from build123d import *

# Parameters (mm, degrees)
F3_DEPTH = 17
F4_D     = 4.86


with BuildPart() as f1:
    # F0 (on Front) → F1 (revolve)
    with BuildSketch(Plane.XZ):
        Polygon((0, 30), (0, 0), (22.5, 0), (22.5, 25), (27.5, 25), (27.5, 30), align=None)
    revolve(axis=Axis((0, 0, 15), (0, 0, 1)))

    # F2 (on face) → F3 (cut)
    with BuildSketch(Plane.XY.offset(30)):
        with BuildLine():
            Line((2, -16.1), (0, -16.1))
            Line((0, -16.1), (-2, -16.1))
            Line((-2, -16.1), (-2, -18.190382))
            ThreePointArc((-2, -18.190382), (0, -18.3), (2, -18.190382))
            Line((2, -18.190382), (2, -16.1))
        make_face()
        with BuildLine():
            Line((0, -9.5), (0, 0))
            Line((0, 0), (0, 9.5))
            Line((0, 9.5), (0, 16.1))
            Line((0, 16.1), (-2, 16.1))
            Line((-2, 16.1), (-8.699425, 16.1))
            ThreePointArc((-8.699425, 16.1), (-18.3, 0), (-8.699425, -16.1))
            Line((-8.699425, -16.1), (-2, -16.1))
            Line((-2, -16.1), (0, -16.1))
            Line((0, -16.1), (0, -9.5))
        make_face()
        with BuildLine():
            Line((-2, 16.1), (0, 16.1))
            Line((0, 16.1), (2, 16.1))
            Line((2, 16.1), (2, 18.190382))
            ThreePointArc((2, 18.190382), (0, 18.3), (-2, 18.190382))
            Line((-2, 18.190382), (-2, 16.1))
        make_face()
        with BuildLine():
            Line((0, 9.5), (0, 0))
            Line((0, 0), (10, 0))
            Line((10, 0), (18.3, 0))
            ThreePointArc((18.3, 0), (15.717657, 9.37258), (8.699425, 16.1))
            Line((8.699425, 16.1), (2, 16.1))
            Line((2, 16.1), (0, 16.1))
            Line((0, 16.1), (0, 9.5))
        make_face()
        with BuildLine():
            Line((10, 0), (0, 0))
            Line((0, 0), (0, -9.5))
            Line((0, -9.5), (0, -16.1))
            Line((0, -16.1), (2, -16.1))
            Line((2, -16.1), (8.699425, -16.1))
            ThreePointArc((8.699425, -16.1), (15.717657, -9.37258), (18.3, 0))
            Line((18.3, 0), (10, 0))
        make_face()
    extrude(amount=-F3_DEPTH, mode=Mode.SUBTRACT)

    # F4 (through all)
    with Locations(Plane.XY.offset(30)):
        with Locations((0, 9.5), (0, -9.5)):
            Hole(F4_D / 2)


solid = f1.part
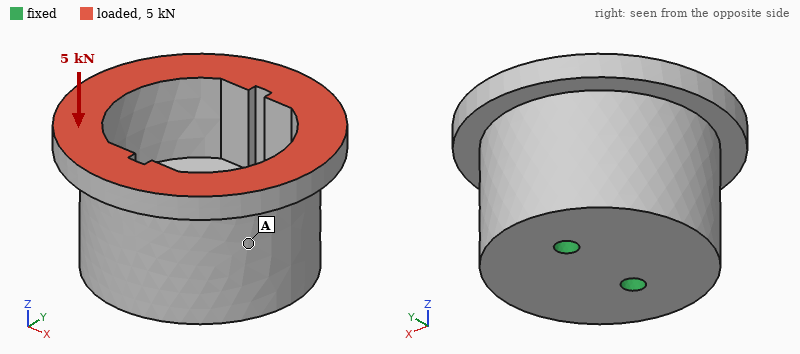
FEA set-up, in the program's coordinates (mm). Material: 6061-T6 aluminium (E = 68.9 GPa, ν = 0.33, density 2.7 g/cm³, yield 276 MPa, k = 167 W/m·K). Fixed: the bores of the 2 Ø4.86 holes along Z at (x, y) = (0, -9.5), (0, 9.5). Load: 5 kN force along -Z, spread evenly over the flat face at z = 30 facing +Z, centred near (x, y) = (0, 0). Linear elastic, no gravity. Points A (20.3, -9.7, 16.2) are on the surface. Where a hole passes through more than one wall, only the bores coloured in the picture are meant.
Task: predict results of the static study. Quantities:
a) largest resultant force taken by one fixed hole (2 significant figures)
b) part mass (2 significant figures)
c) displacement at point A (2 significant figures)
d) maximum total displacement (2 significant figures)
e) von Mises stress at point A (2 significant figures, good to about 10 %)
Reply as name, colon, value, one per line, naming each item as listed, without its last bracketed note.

largest resultant force taken by one fixed hole: 2.5 kN
part mass: 91 g
displacement at point A: 6.6 µm
maximum total displacement: 15 µm
von Mises stress at point A: 6.3 MPa
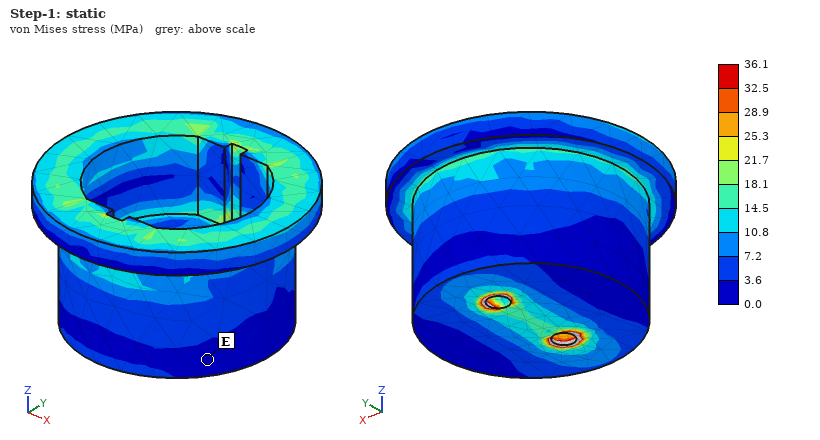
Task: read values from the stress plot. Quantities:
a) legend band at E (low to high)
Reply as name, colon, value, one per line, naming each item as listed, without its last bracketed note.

legend band at E: 0.0 to 3.6 MPa
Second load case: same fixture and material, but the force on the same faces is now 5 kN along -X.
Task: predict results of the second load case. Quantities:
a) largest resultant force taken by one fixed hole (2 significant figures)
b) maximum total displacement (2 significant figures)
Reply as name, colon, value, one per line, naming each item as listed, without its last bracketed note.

largest resultant force taken by one fixed hole: 2.5 kN
maximum total displacement: 72 µm
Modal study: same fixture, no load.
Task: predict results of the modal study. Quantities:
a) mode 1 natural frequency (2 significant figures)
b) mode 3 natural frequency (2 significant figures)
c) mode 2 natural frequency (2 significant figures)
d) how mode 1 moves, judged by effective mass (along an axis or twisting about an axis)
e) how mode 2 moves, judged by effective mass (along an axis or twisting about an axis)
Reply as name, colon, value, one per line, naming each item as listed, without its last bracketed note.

mode 1 natural frequency: 8800 Hz
mode 3 natural frequency: 13 kHz
mode 2 natural frequency: 12 kHz
how mode 1 moves, judged by effective mass: along X
how mode 2 moves, judged by effective mass: along Y
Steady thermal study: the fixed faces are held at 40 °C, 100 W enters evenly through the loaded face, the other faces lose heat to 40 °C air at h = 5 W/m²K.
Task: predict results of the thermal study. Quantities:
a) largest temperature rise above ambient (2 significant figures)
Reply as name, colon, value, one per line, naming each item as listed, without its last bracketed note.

largest temperature rise above ambient: 28 K
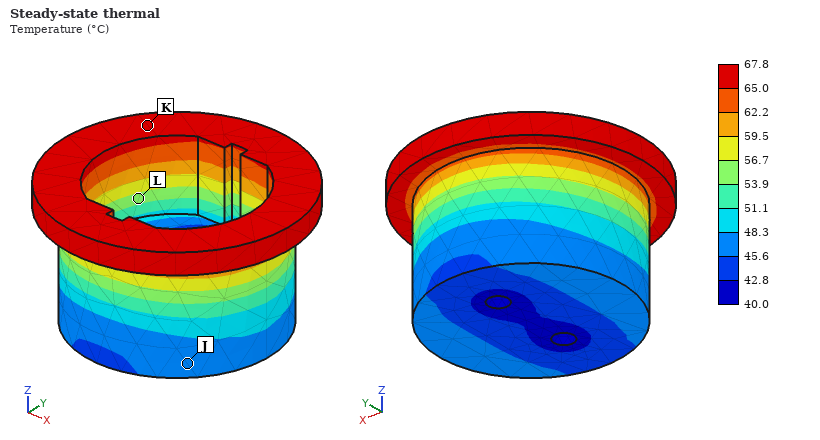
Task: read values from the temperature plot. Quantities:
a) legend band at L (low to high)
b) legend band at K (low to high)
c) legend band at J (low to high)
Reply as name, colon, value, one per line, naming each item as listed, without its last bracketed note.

legend band at L: 53.9 to 56.7 °C
legend band at K: 65.0 to 67.8 °C
legend band at J: 45.6 to 48.3 °C
